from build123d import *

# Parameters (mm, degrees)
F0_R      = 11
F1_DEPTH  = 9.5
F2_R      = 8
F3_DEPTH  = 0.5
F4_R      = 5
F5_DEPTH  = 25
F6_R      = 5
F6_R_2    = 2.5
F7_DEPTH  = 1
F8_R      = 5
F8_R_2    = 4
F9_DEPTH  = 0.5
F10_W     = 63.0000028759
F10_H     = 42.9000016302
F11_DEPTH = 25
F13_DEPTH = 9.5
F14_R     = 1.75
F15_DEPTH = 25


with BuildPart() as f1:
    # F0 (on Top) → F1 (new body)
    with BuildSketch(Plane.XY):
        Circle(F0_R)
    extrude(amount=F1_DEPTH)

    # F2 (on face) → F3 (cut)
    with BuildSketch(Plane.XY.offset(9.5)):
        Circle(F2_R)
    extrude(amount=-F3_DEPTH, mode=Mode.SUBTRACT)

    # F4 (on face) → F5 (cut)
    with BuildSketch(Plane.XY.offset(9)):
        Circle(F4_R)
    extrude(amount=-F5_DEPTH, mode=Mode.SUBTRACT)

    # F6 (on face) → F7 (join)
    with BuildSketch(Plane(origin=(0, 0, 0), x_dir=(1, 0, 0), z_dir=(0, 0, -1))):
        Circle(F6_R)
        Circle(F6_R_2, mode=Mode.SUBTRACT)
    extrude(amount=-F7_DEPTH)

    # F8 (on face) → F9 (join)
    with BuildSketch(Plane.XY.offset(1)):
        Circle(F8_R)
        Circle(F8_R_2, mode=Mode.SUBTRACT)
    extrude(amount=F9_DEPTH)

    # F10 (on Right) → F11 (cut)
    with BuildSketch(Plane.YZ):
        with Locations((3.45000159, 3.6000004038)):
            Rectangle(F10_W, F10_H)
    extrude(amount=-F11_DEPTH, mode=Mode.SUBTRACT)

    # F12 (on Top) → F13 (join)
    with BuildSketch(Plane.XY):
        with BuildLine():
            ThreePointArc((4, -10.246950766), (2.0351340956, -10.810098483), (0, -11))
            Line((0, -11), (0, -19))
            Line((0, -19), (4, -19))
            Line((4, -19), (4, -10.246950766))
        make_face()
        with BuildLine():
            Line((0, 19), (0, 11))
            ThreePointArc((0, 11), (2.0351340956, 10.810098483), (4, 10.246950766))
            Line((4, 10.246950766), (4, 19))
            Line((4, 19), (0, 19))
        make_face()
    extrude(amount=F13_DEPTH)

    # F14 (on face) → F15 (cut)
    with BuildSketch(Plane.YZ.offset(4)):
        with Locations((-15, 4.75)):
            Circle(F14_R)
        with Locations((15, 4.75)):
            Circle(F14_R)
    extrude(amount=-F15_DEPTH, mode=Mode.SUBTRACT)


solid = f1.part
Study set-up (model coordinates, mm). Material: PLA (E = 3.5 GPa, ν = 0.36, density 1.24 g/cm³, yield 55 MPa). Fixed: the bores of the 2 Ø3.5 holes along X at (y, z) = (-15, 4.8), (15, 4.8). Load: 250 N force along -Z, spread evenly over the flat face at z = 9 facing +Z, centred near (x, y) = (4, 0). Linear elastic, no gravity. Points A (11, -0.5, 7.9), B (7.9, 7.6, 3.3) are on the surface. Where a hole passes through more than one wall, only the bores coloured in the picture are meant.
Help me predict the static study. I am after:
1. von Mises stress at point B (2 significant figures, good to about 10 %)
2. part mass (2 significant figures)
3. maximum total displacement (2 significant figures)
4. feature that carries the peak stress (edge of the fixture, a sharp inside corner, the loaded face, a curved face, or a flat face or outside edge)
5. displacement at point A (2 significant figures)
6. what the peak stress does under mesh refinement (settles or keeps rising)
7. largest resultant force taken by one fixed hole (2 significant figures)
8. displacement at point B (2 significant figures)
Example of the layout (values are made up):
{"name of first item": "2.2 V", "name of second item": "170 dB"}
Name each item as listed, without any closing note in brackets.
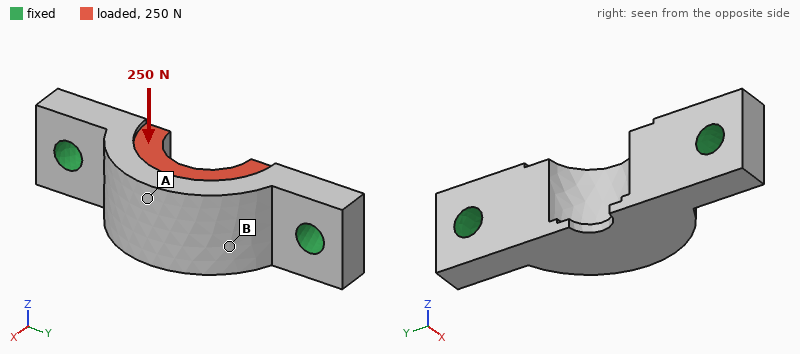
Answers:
{"von Mises stress at point B": "6.6 MPa", "part mass": "2.5 g", "maximum total displacement": "0.13 mm", "feature that carries the peak stress": "edge of the fixture", "displacement at point A": "0.13 mm", "what the peak stress does under mesh refinement": "keeps rising", "largest resultant force taken by one fixed hole": "130 N", "displacement at point B": "0.085 mm"}
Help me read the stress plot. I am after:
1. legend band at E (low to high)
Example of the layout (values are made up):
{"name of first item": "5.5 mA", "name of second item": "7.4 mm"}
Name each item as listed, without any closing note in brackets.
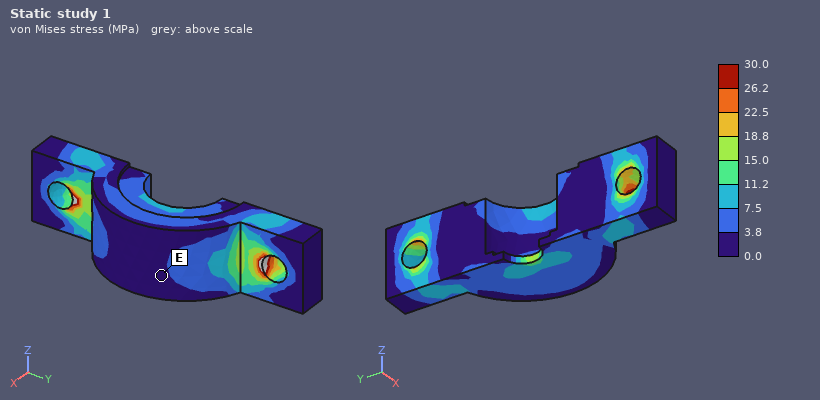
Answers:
{"legend band at E": "0.0 to 3.8 MPa"}
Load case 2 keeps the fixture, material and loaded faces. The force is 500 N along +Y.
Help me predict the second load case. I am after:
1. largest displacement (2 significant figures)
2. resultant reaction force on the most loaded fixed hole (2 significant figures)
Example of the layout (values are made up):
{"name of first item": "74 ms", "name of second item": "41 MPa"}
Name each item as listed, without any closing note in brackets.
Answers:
{"largest displacement": "49 µm", "resultant reaction force on the most loaded fixed hole": "260 N"}
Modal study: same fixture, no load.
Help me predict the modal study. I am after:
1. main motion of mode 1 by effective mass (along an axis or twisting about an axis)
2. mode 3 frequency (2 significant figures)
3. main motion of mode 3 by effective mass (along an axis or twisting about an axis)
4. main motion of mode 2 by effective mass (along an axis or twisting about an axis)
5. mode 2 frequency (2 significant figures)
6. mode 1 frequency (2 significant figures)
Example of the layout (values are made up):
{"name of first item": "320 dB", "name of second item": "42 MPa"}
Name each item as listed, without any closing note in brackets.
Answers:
{"main motion of mode 1 by effective mass": "along Z", "mode 3 frequency": "14 kHz", "main motion of mode 3 by effective mass": "along Z", "main motion of mode 2 by effective mass": "along X", "mode 2 frequency": "9500 Hz", "mode 1 frequency": "5600 Hz"}
